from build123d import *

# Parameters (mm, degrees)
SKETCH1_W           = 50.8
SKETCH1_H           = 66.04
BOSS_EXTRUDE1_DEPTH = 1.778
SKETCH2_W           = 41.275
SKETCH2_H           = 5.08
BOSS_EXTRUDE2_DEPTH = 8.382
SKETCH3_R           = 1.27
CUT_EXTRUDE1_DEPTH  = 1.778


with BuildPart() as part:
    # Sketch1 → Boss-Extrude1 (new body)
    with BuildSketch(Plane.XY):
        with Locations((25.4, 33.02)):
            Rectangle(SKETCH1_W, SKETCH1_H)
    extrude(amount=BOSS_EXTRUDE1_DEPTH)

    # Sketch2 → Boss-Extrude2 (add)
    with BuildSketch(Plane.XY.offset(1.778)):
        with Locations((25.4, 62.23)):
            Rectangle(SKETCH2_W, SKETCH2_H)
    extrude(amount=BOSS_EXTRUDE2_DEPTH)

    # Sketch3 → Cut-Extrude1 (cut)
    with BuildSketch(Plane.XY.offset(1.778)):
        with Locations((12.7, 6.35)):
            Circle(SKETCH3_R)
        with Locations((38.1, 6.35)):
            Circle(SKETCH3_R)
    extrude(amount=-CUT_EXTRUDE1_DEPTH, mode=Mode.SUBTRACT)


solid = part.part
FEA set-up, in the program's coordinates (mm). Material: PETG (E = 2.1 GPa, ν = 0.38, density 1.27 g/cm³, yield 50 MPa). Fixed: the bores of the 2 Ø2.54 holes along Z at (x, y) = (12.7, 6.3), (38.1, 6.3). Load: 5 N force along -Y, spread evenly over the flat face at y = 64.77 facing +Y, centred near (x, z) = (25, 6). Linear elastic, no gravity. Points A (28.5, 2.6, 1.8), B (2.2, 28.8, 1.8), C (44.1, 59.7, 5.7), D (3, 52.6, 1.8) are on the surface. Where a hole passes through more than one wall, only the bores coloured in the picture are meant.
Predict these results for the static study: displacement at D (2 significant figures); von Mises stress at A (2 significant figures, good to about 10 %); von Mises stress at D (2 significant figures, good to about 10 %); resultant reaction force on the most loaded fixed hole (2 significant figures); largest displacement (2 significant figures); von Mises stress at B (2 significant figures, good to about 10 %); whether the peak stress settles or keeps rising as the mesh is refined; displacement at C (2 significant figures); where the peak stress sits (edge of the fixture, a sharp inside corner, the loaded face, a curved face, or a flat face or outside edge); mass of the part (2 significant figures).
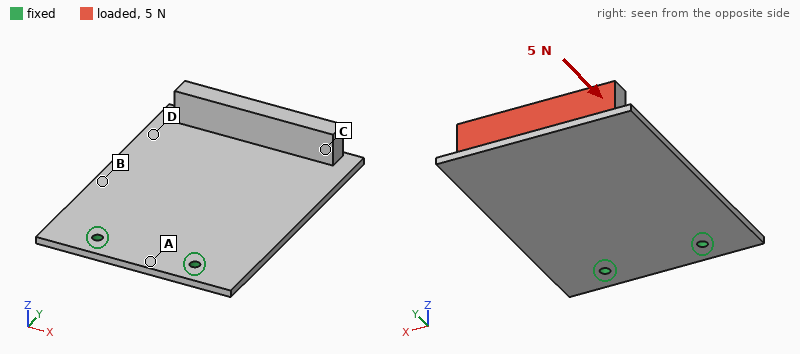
0.54 mm
0.26 MPa
0.89 MPa
2.5 N
0.89 mm
1.0 MPa
keeps rising
0.73 mm
edge of the fixture
9.8 g
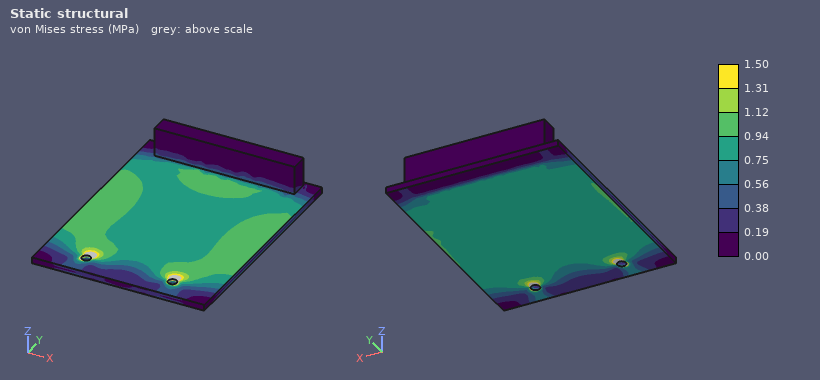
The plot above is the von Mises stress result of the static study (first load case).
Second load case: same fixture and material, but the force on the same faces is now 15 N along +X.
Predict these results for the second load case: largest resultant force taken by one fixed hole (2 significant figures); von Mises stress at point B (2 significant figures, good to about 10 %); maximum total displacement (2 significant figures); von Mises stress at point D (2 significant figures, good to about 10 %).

34 N
1.9 MPa
0.93 mm
2.1 MPa
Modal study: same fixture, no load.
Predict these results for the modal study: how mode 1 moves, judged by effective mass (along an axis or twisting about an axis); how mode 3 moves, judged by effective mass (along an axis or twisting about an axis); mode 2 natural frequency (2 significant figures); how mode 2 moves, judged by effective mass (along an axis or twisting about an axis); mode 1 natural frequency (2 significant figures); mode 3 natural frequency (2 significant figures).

along Z
along Z
230 Hz
twisting about Y
70 Hz
510 Hz
